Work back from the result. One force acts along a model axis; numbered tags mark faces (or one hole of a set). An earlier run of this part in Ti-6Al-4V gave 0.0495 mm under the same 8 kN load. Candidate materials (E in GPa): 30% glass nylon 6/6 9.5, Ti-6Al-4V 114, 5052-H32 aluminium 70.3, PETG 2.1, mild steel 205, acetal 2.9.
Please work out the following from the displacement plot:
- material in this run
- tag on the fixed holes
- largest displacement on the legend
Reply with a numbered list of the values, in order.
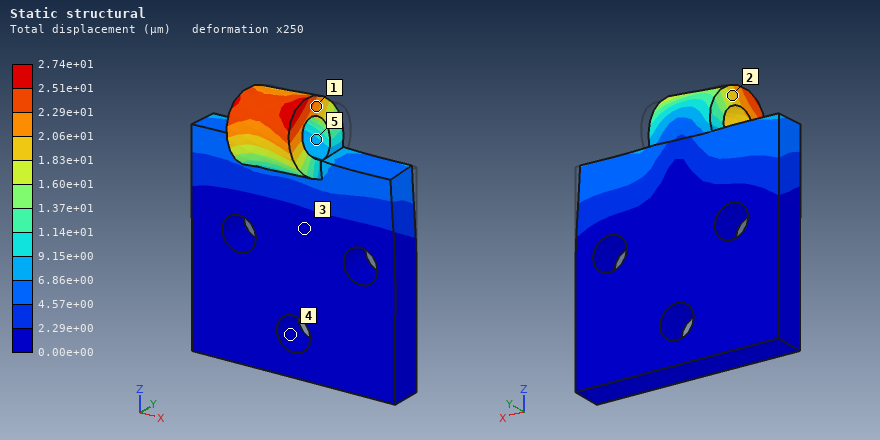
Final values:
1. mild steel
2. 4
3. 2.74e+01 µm
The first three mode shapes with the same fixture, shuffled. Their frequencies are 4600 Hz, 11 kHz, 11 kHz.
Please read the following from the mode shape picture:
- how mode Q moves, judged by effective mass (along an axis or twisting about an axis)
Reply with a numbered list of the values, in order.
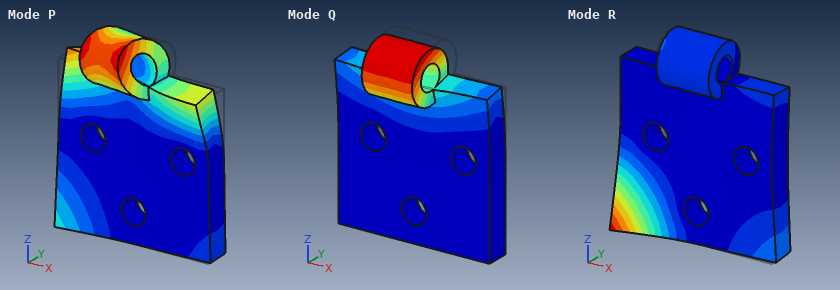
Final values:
1. along Y
